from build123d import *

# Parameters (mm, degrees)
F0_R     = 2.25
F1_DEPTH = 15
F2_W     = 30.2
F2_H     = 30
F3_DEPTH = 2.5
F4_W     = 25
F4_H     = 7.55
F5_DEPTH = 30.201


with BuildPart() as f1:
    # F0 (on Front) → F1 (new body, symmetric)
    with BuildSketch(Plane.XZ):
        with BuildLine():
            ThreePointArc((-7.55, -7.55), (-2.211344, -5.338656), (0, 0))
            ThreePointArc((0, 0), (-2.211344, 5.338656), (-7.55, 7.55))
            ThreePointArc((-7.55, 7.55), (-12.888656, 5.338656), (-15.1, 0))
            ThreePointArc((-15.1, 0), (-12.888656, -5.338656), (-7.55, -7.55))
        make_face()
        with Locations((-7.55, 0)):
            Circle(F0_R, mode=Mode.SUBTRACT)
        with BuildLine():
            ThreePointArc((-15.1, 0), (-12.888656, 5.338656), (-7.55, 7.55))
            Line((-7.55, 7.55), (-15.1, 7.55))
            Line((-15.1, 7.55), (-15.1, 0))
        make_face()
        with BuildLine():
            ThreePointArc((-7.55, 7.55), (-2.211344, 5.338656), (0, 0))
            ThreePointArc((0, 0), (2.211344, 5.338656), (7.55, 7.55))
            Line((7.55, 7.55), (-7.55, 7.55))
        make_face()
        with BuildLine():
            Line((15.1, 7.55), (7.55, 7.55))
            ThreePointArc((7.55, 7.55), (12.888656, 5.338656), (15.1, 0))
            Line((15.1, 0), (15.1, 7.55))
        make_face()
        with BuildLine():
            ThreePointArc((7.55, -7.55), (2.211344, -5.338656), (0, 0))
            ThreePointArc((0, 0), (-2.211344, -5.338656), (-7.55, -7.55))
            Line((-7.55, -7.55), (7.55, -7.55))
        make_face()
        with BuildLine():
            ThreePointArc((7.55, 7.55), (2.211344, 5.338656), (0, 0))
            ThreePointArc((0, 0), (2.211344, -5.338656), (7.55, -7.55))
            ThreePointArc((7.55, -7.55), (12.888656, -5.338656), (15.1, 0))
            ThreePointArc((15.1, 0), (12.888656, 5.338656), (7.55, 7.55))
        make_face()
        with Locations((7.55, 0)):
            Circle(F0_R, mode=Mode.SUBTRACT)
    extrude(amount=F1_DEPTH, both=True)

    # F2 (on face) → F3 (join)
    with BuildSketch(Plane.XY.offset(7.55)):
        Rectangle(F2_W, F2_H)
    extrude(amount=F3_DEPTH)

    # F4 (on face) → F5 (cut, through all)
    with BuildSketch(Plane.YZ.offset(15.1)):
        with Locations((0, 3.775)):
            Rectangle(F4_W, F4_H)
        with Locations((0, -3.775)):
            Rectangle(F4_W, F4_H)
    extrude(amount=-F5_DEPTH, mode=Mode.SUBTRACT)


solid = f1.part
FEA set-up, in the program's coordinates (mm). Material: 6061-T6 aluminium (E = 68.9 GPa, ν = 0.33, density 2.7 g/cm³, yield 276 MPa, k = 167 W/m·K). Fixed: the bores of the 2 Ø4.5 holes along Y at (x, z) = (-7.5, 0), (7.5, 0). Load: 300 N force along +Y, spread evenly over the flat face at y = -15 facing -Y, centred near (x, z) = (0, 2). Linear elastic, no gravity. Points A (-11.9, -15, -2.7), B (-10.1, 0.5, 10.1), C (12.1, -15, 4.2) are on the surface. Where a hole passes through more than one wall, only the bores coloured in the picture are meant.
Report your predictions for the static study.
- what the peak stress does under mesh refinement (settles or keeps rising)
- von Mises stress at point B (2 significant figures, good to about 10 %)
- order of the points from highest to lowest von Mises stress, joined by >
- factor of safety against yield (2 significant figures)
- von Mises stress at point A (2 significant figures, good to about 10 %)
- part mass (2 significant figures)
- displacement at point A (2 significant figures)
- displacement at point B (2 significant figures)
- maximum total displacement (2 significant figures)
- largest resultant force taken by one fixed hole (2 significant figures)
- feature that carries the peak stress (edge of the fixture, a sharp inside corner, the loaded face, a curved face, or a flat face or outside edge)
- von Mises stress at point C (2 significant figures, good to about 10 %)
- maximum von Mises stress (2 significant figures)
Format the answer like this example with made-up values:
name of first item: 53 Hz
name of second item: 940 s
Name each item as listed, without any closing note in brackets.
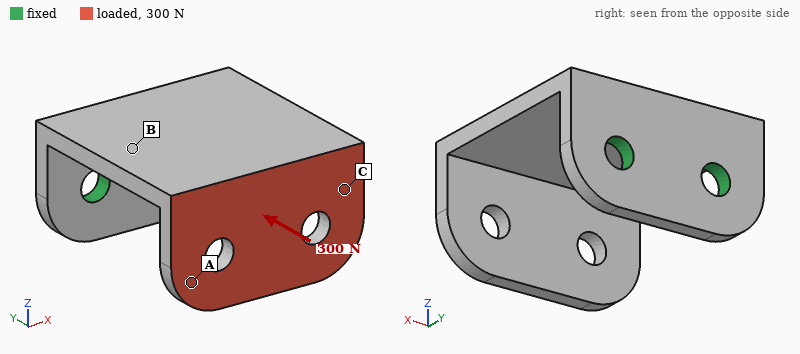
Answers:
what the peak stress does under mesh refinement: settles
von Mises stress at point B: 61 MPa
order of the points from highest to lowest von Mises stress, joined by >: B > C > A
factor of safety against yield: 3.8
von Mises stress at point A: 9.8 MPa
part mass: 12 g
displacement at point A: 0.45 mm
displacement at point B: 0.089 mm
maximum total displacement: 0.54 mm
largest resultant force taken by one fixed hole: 150 N
feature that carries the peak stress: a flat face or outside edge
von Mises stress at point C: 32 MPa
maximum von Mises stress: 72 MPa
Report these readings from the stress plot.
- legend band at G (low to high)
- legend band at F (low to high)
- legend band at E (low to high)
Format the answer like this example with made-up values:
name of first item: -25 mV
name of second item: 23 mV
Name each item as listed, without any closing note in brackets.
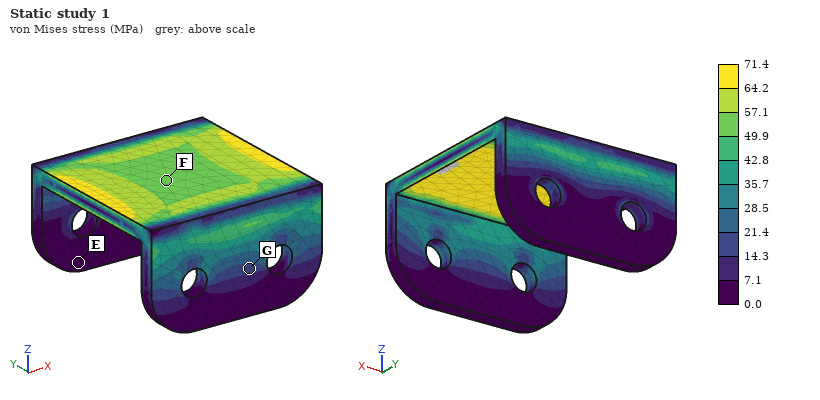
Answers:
legend band at G: 14.3 to 21.4 MPa
legend band at F: 49.9 to 57.1 MPa
legend band at E: 0.0 to 7.1 MPa
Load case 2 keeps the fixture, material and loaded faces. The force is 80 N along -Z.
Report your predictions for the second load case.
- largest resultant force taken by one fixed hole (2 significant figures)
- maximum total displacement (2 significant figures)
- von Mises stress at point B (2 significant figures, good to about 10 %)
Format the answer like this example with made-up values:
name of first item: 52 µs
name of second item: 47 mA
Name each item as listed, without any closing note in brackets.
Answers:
largest resultant force taken by one fixed hole: 44 N
maximum total displacement: 0.45 mm
von Mises stress at point B: 38 MPa
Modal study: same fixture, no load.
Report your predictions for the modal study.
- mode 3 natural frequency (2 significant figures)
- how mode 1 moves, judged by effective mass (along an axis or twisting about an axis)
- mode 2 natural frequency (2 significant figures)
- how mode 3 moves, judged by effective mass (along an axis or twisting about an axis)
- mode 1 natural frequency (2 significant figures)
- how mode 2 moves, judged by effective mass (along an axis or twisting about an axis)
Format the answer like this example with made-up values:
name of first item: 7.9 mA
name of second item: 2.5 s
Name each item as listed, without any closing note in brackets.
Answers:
mode 3 natural frequency: 4300 Hz
how mode 1 moves, judged by effective mass: along Z
mode 2 natural frequency: 2400 Hz
how mode 3 moves, judged by effective mass: along Y
mode 1 natural frequency: 1100 Hz
how mode 2 moves, judged by effective mass: along X
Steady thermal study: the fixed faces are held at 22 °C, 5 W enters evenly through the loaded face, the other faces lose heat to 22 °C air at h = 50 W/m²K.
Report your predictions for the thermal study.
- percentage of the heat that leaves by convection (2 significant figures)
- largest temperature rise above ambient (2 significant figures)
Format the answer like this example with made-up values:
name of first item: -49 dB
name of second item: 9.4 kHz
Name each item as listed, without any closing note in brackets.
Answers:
percentage of the heat that leaves by convection: 21 %
largest temperature rise above ambient: 14 K
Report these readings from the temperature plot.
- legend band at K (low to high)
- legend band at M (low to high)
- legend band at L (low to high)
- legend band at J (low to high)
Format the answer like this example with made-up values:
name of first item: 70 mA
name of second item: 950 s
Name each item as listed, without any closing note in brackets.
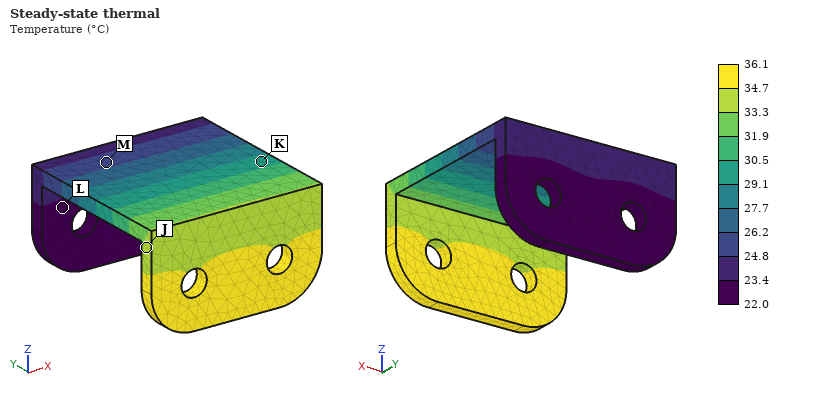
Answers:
legend band at K: 29.1 to 30.5 °C
legend band at M: 24.8 to 26.2 °C
legend band at L: 22.0 to 23.4 °C
legend band at J: 33.3 to 34.7 °C
